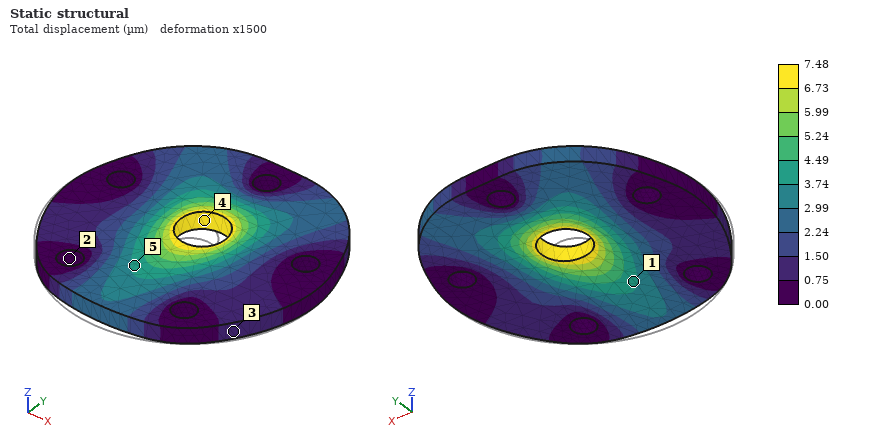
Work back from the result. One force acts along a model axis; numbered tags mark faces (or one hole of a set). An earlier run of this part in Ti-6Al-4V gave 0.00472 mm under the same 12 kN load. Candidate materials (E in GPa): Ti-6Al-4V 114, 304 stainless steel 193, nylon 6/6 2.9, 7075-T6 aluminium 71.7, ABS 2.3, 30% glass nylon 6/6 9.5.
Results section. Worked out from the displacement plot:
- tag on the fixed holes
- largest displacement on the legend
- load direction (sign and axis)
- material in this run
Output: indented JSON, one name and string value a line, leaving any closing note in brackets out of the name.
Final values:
{
  "tag on the fixed holes": "2",
  "largest displacement on the legend": "7.48 µm",
  "load direction": "+Y",
  "material in this run": "7075-T6 aluminium"
}
